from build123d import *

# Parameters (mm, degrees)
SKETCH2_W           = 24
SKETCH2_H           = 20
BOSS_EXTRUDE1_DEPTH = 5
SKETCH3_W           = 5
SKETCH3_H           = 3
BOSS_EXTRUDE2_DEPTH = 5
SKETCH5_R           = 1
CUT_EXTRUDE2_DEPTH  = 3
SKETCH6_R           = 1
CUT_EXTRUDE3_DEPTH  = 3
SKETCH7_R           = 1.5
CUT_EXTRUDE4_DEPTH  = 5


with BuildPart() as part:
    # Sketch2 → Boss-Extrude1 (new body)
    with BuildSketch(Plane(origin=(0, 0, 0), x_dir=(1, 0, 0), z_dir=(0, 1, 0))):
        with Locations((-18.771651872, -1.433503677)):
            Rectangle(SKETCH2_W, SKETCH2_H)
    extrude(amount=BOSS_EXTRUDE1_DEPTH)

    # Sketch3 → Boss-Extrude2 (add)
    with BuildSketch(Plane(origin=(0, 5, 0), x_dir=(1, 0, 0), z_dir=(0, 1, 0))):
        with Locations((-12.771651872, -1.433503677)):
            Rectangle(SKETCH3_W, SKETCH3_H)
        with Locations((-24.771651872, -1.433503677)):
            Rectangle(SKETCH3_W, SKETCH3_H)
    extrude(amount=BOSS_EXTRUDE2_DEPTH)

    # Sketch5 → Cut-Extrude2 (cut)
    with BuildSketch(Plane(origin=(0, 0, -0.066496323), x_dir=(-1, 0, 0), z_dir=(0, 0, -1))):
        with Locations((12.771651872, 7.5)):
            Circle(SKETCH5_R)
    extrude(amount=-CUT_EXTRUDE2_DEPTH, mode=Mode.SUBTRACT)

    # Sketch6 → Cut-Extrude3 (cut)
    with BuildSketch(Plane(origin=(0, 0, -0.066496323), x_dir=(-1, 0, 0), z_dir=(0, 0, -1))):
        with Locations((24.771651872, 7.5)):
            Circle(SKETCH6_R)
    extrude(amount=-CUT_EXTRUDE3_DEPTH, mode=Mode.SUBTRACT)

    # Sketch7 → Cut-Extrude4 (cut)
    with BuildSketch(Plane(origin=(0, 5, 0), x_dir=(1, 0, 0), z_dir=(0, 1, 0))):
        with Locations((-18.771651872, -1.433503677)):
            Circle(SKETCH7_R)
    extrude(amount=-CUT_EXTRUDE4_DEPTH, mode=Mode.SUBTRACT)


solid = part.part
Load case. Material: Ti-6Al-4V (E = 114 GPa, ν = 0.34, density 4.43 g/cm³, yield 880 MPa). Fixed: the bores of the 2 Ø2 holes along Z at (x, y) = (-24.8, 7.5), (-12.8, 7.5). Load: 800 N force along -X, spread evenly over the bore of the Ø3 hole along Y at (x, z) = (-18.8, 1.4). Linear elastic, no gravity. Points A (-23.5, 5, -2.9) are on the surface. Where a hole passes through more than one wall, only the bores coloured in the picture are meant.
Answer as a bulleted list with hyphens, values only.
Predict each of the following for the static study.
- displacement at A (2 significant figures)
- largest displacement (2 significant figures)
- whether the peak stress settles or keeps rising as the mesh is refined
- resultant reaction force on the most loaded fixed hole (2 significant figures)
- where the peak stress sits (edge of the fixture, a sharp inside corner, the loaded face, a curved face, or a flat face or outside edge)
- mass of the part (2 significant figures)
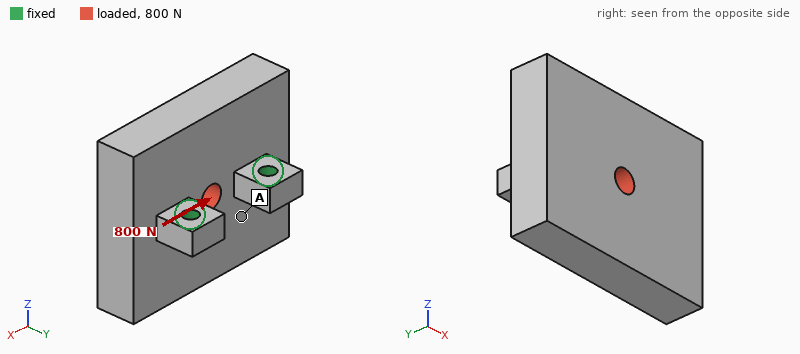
- 2.7 µm
- 4.0 µm
- keeps rising
- 460 N
- edge of the fixture
- 11 g
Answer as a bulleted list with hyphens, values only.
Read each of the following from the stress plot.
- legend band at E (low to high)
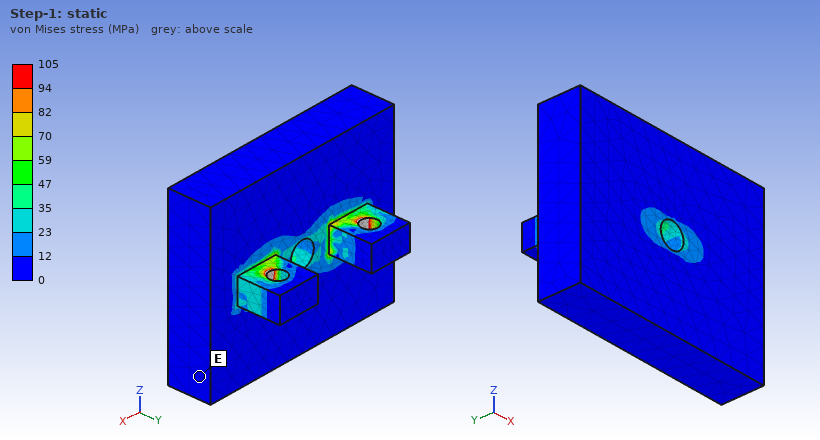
- 0 to 12 MPa
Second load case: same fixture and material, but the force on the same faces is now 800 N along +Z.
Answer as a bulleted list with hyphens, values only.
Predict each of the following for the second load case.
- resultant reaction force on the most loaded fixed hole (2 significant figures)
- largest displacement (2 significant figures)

- 400 N
- 35 µm
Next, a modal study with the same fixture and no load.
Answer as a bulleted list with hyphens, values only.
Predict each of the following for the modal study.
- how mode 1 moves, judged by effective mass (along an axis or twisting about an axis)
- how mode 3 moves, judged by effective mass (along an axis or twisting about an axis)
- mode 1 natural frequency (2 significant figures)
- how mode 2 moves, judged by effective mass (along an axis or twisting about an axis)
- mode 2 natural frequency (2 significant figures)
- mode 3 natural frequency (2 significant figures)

- along Z
- along X
- 6700 Hz
- twisting about Y
- 16 kHz
- 23 kHz
